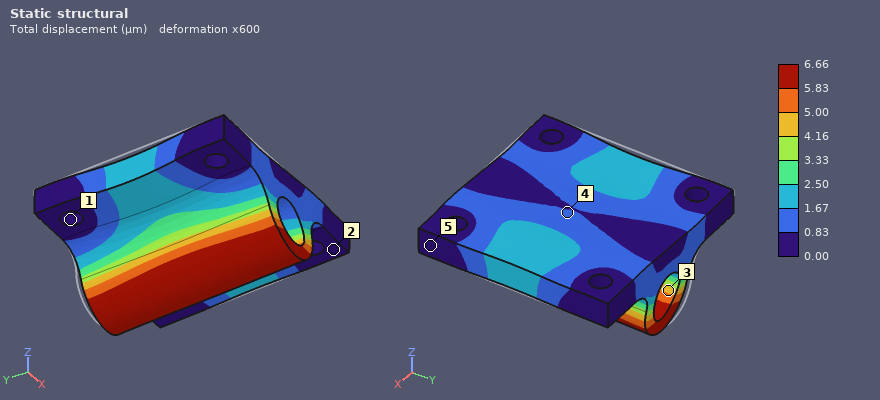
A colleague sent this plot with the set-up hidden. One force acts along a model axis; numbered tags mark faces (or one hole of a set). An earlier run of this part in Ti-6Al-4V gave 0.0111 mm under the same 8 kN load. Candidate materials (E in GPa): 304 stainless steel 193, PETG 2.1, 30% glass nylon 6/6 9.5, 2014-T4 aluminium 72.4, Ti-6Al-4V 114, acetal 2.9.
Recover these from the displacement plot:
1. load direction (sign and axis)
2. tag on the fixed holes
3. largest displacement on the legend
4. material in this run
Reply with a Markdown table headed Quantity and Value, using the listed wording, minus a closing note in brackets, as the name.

| Quantity | Value |
|---|---|
| load direction | +X |
| tag on the fixed holes | 1 |
| largest displacement on the legend | 6.66 µm |
| material in this run | 304 stainless steel |
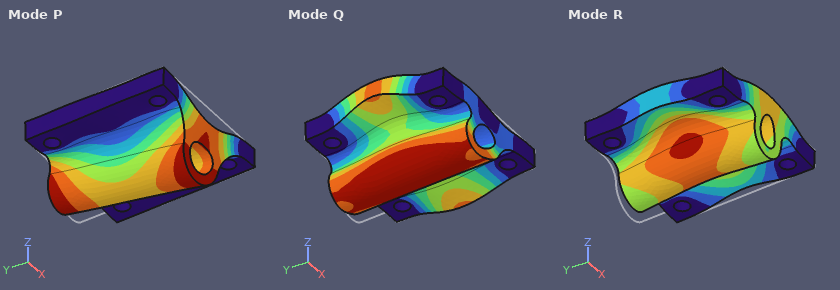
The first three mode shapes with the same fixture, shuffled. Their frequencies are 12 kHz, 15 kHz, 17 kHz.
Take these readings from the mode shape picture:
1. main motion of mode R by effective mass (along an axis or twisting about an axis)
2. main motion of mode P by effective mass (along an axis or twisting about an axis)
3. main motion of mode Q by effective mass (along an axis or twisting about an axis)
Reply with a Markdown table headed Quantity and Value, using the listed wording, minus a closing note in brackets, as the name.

| Quantity | Value |
|---|---|
| main motion of mode R by effective mass | along Z |
| main motion of mode P by effective mass | along Y |
| main motion of mode Q by effective mass | along X |
